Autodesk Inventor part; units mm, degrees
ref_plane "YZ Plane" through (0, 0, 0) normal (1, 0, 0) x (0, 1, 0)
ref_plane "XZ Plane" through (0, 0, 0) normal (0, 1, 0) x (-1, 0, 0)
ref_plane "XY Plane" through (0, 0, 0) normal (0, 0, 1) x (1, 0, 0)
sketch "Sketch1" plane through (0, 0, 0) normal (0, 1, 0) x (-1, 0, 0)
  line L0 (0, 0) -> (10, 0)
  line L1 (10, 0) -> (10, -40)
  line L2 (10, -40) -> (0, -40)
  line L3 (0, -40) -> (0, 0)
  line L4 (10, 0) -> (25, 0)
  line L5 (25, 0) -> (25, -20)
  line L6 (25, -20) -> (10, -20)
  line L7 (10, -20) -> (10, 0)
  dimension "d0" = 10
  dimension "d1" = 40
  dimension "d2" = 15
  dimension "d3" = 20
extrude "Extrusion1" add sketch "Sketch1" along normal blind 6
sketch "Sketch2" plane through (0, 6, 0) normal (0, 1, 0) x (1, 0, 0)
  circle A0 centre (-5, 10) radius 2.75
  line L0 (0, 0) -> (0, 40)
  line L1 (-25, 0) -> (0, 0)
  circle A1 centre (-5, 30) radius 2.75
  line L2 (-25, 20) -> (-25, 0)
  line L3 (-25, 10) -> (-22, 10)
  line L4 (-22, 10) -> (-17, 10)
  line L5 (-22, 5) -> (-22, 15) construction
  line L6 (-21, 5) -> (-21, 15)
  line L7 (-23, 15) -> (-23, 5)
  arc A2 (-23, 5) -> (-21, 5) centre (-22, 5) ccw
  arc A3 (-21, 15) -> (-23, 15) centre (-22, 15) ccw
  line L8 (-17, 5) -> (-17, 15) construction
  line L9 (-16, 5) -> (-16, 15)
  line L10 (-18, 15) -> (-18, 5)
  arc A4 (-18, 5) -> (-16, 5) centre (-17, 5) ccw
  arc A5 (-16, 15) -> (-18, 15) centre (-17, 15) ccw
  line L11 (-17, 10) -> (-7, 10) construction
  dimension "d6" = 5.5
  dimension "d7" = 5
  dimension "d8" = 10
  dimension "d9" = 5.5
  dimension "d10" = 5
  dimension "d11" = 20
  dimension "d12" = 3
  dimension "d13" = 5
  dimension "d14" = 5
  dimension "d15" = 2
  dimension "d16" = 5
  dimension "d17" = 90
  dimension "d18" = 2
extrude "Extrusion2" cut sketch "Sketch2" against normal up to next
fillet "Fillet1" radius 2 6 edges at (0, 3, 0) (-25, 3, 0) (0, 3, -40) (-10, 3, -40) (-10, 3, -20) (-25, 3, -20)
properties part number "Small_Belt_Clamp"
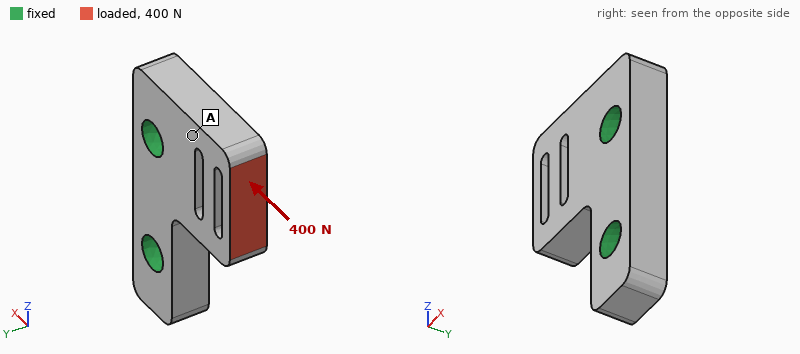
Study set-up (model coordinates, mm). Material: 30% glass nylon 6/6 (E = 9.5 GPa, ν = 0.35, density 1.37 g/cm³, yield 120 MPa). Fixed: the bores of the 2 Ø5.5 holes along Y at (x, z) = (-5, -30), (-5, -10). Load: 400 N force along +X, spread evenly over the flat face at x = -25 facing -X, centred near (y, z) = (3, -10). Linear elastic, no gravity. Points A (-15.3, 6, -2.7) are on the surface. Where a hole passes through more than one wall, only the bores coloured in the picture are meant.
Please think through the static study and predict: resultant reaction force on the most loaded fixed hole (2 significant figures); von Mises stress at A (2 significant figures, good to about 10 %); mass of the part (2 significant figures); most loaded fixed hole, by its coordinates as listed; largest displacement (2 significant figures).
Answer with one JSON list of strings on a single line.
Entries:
["370 N", "9.1 MPa", "5.0 g", "(-5, -10)", "93 µm"]
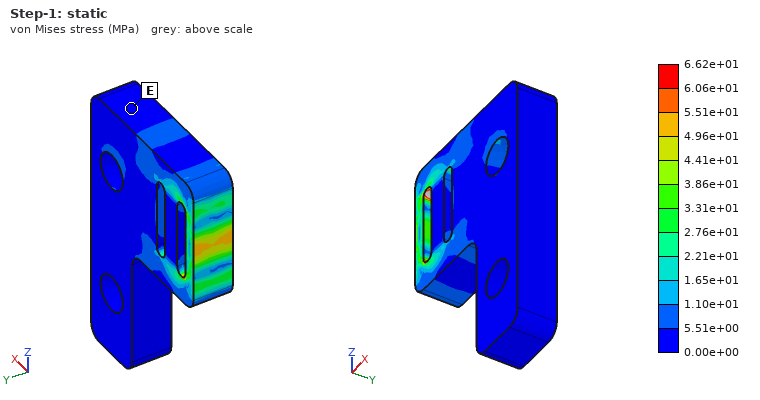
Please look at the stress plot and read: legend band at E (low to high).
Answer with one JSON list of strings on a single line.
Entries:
["0.00e+00 to 5.51e+00 MPa"]
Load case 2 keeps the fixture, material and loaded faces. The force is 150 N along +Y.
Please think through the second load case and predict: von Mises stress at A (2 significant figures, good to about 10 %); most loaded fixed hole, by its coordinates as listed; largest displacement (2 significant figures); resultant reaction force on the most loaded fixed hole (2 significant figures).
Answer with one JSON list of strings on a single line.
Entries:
["28 MPa", "(-5, -10)", "0.18 mm", "160 N"]
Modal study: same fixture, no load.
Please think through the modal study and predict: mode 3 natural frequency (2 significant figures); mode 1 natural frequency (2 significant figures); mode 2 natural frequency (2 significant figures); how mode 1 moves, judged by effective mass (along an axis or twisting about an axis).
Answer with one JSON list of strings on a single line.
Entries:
["11 kHz", "6500 Hz", "10 kHz", "along Y"]
